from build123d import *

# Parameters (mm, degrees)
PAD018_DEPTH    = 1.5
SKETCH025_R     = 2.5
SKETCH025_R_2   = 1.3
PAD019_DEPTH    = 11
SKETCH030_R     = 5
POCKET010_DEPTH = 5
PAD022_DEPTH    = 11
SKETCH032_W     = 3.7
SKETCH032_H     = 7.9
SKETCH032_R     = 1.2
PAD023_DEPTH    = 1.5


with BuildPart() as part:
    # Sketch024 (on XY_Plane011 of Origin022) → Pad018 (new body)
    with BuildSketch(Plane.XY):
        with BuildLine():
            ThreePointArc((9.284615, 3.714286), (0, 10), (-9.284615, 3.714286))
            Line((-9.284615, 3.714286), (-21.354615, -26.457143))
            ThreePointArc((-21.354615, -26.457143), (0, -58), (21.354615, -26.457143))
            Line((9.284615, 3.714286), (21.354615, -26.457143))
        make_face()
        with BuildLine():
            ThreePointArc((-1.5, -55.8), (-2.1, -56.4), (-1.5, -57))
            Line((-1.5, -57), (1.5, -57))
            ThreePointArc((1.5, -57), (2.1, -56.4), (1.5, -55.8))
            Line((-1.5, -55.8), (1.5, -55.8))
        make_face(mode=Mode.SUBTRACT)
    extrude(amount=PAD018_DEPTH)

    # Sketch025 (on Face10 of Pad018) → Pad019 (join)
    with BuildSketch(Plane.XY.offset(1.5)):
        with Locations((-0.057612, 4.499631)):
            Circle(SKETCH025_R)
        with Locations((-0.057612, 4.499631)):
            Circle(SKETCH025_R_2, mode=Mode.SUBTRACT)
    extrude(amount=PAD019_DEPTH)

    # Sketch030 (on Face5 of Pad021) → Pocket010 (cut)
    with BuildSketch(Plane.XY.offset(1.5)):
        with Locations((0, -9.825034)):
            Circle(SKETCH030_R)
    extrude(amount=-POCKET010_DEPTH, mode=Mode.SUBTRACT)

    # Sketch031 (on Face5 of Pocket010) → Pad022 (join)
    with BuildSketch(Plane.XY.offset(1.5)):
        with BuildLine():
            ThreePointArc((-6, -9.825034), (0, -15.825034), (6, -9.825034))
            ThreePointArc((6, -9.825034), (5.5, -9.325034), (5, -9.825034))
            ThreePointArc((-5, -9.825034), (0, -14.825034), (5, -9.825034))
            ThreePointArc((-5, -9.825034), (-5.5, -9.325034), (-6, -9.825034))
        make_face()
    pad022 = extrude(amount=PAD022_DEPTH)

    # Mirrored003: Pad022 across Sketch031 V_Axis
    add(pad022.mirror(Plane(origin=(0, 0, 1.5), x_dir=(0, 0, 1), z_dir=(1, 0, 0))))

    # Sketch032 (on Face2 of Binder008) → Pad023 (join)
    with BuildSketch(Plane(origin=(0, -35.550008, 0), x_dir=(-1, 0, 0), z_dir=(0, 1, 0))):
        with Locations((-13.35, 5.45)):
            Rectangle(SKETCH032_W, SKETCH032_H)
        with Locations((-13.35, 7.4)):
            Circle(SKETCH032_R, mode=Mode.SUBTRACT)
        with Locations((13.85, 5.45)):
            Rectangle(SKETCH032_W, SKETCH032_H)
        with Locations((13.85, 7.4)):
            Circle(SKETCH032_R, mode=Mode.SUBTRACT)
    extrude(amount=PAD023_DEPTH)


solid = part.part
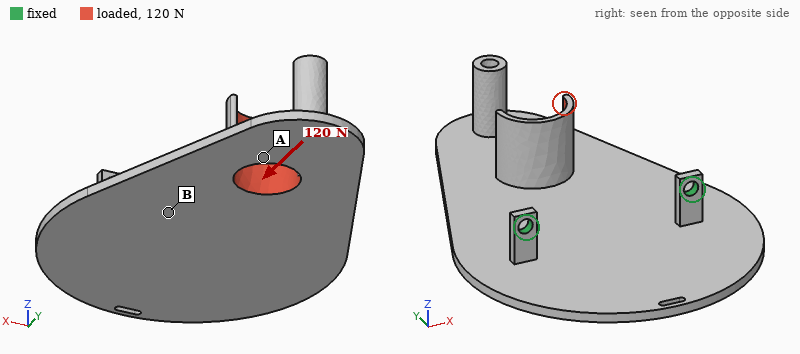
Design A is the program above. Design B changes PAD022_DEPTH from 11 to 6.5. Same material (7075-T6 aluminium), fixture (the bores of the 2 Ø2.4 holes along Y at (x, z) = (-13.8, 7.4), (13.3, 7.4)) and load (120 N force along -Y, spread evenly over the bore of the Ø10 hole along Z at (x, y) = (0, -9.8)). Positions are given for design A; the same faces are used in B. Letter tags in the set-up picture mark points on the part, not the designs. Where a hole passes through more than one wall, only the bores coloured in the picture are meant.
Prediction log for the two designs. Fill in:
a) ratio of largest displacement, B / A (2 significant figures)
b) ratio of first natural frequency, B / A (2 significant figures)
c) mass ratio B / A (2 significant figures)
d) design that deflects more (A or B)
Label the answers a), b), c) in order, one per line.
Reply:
a) 0.28
b) 1.0
c) 0.98
d) A
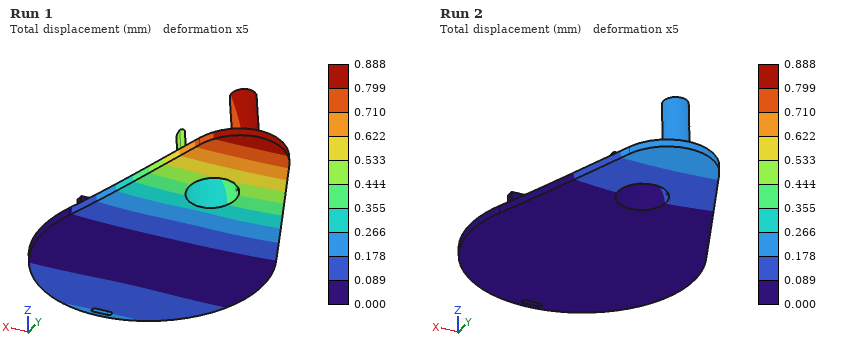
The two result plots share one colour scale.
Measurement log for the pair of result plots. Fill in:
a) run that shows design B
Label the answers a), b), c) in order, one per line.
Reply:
a) Run 2
